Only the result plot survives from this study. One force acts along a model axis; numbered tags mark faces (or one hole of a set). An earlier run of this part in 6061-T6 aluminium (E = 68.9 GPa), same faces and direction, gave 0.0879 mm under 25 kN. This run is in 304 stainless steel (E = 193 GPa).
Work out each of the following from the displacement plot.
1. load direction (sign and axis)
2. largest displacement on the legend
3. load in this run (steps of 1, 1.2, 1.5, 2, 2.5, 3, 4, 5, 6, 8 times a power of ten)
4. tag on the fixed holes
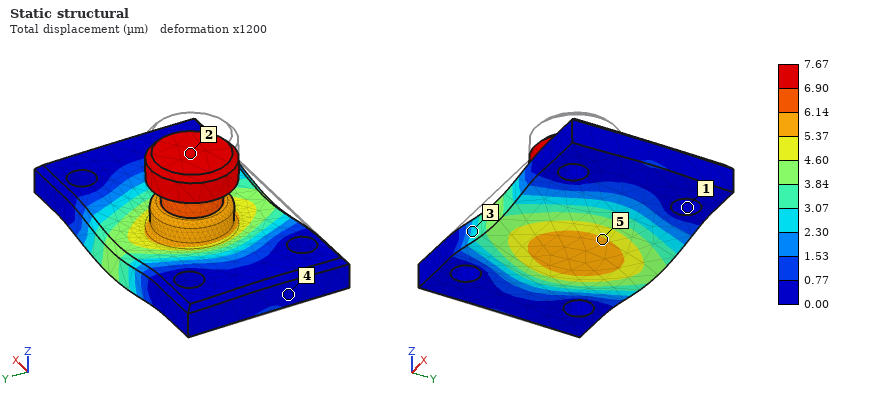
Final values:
-Z
7.67 µm
6 kN
1
